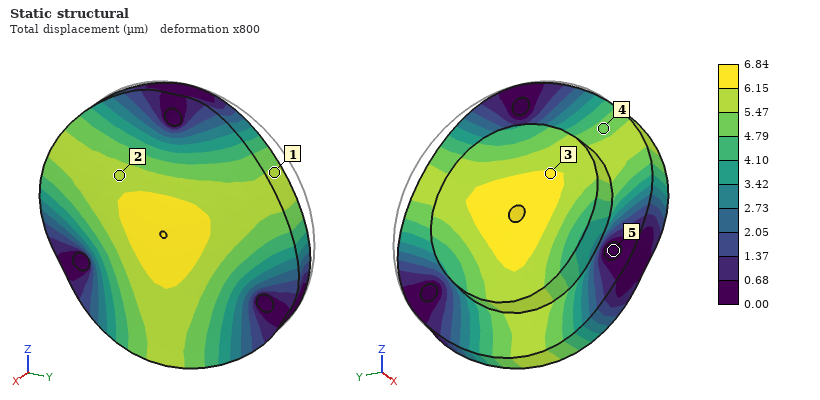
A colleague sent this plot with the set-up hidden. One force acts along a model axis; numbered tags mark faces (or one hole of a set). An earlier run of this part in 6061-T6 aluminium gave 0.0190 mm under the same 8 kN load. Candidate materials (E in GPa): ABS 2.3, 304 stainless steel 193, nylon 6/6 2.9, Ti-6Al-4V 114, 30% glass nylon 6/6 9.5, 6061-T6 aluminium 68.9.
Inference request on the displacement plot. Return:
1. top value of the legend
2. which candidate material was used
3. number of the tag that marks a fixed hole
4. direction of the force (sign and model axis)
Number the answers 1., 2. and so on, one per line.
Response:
1. 6.84 µm
2. 304 stainless steel
3. 5
4. +X
